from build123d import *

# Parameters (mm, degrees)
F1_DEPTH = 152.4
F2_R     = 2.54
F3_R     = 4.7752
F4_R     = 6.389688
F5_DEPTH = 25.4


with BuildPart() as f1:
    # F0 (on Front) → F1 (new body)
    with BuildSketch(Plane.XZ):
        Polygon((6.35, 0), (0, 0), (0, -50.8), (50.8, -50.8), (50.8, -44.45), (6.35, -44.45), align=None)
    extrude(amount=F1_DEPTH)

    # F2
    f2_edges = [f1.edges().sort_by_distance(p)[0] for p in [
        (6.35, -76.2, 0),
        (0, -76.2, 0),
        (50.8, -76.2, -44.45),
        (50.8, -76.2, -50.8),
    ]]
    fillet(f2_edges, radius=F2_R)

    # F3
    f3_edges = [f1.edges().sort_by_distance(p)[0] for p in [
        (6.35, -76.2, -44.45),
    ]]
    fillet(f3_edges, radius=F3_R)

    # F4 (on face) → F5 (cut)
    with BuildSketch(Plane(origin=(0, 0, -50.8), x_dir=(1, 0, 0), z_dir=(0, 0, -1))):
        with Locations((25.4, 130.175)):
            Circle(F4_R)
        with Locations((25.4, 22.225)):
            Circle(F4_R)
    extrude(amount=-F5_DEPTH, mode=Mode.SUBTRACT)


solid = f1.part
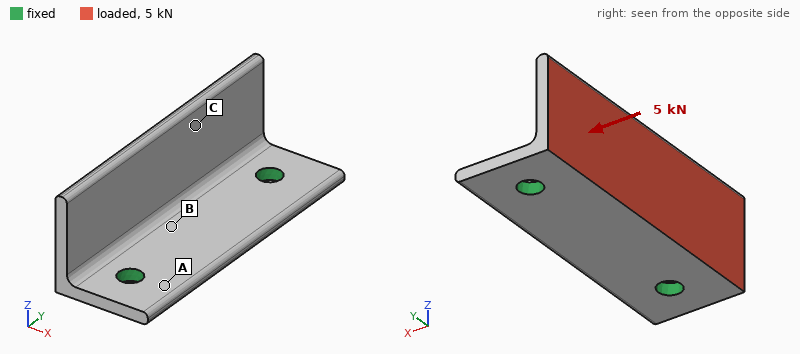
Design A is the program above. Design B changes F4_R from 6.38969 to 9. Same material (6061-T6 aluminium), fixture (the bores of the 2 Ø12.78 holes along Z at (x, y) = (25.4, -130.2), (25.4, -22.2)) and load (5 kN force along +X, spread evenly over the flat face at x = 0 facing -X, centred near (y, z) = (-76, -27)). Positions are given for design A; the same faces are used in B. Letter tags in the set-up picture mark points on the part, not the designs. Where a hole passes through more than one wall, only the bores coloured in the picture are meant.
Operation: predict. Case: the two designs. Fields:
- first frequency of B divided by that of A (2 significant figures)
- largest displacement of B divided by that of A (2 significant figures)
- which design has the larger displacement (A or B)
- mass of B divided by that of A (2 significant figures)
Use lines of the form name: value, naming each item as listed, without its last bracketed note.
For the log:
first frequency of B divided by that of A: 1.1
largest displacement of B divided by that of A: 0.85
which design has the larger displacement: A
mass of B divided by that of A: 0.98
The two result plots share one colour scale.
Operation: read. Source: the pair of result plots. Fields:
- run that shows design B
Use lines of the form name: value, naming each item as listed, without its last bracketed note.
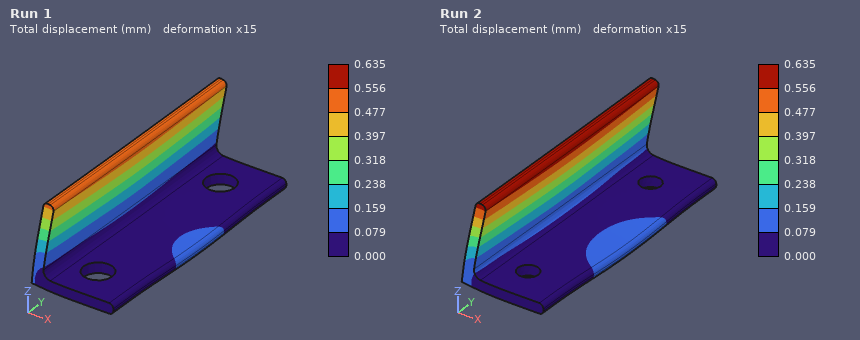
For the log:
run that shows design B: Run 1
